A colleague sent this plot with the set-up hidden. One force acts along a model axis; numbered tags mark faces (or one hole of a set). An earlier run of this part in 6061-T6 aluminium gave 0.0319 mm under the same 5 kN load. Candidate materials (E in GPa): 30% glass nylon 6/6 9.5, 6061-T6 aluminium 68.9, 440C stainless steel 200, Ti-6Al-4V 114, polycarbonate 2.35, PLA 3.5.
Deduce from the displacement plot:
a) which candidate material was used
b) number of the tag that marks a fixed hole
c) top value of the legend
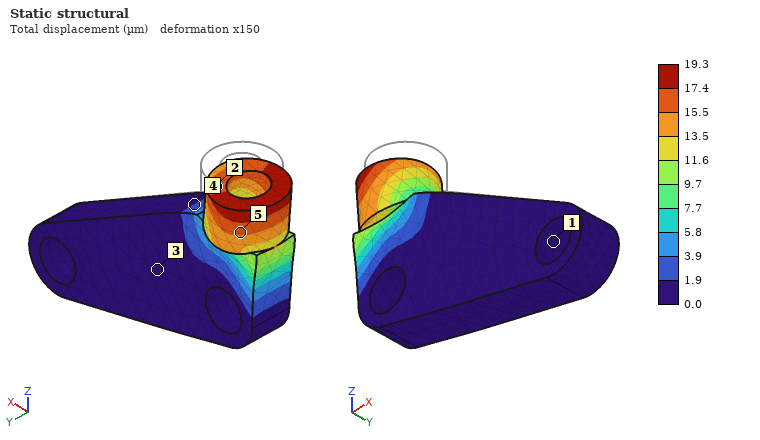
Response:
Ti-6Al-4V
1
19.3 µm
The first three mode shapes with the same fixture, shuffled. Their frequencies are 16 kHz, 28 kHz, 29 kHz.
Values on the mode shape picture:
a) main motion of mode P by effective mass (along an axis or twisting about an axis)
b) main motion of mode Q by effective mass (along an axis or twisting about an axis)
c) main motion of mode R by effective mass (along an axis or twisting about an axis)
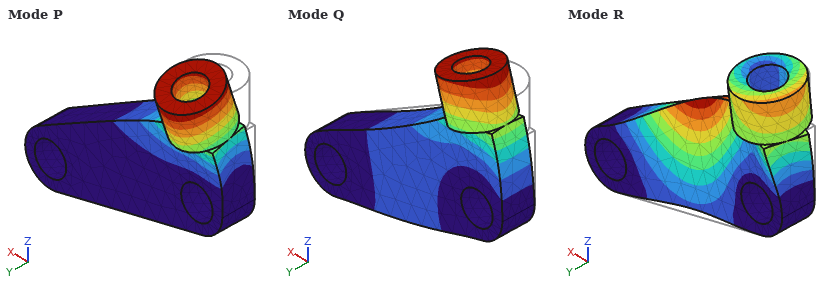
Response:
along Y
along X
along Y
